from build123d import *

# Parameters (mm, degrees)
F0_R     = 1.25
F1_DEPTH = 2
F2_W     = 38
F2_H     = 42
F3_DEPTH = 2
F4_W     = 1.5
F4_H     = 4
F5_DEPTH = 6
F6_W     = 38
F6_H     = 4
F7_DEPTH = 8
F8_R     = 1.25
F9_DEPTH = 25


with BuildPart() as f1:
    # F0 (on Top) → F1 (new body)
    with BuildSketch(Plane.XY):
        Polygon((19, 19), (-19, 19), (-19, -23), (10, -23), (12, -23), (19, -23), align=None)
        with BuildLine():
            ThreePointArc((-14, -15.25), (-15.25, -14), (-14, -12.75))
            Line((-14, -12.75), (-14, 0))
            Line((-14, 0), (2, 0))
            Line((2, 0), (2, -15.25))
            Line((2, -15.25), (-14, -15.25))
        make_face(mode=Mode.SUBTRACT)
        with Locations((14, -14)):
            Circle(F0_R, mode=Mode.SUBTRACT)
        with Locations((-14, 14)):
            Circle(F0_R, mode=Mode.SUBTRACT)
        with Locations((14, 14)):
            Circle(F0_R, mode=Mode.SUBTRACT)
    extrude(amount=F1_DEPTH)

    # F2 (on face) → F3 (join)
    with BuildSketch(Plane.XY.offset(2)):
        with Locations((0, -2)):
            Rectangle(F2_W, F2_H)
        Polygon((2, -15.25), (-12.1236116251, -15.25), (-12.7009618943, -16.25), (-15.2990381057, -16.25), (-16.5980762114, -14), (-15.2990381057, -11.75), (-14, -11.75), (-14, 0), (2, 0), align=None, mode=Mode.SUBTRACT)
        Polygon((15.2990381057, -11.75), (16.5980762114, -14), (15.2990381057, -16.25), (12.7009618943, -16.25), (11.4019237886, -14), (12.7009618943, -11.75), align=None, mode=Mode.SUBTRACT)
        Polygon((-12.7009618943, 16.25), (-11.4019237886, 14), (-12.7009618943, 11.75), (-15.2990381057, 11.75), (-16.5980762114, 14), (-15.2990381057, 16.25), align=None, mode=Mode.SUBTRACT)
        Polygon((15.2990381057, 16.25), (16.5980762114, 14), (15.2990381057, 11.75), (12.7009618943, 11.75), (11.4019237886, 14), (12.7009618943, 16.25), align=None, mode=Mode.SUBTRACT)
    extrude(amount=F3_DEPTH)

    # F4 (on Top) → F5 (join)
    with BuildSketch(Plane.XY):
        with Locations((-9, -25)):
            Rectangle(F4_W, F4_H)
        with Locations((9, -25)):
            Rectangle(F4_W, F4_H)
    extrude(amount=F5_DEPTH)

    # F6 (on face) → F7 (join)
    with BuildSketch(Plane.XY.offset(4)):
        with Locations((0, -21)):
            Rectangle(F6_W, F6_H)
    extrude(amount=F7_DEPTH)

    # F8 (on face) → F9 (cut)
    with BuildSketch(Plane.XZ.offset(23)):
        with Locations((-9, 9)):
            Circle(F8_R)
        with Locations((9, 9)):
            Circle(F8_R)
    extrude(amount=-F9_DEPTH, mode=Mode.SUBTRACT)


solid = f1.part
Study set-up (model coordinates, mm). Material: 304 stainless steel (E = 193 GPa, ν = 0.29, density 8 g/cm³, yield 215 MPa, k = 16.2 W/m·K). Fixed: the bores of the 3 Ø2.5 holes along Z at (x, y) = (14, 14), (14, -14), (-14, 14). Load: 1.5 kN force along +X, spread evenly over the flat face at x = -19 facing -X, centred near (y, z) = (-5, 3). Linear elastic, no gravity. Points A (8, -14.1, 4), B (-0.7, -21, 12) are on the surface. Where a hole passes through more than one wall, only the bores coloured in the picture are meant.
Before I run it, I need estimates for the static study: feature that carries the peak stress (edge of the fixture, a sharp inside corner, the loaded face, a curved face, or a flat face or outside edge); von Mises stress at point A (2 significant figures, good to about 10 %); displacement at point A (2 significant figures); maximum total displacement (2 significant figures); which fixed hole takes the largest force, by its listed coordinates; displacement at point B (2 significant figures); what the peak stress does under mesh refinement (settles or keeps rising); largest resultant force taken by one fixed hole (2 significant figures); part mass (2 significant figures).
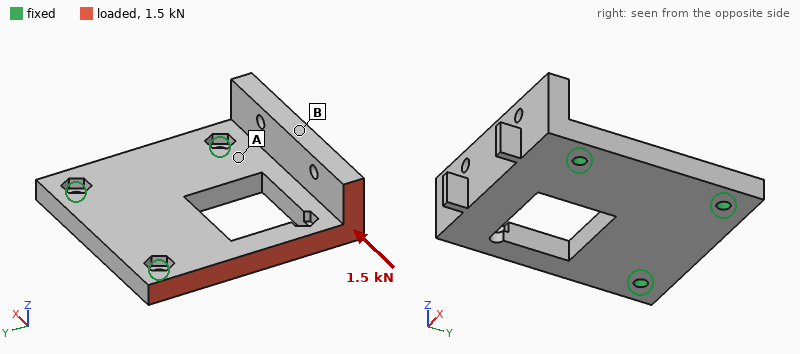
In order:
edge of the fixture
24 MPa
4.2 µm
26 µm
(14, -14)
15 µm
keeps rising
770 N
52 g
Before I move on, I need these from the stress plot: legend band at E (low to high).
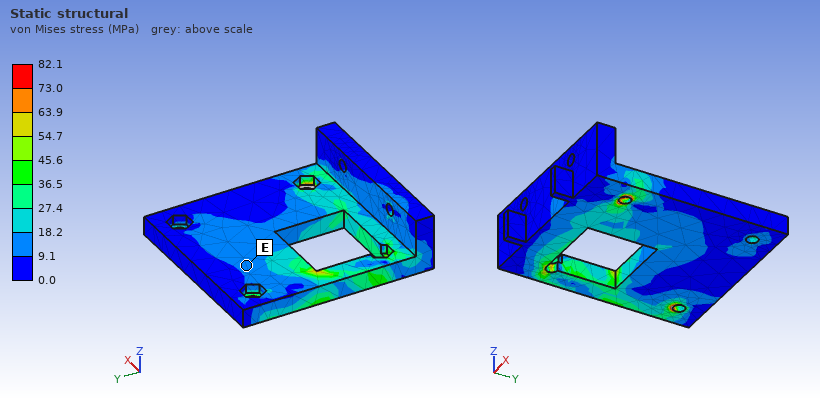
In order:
9.1 to 18.2 MPa
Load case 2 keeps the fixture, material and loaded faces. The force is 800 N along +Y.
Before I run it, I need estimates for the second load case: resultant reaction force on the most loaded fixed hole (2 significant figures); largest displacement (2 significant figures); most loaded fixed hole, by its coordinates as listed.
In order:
770 N
20 µm
(-14, 14)
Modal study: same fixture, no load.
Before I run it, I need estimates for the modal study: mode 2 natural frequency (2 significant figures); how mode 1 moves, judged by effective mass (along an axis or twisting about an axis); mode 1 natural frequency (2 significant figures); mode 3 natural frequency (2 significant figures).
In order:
7900 Hz
along Z
2900 Hz
13 kHz
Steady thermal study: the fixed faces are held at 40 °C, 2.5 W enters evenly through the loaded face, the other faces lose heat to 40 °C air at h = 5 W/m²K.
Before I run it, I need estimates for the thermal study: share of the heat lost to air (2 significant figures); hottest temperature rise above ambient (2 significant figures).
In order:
9.0 %
34 K
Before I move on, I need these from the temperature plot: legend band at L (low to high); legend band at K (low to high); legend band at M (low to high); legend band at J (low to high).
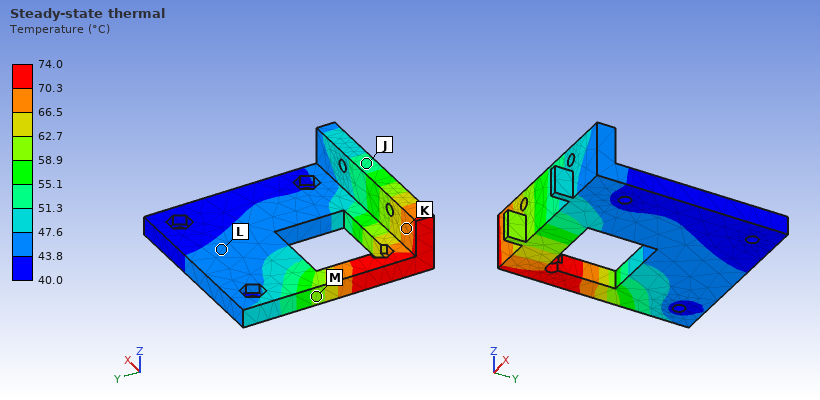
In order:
43.8 to 47.6 °C
66.5 to 70.3 °C
58.9 to 62.7 °C
51.3 to 55.1 °C
